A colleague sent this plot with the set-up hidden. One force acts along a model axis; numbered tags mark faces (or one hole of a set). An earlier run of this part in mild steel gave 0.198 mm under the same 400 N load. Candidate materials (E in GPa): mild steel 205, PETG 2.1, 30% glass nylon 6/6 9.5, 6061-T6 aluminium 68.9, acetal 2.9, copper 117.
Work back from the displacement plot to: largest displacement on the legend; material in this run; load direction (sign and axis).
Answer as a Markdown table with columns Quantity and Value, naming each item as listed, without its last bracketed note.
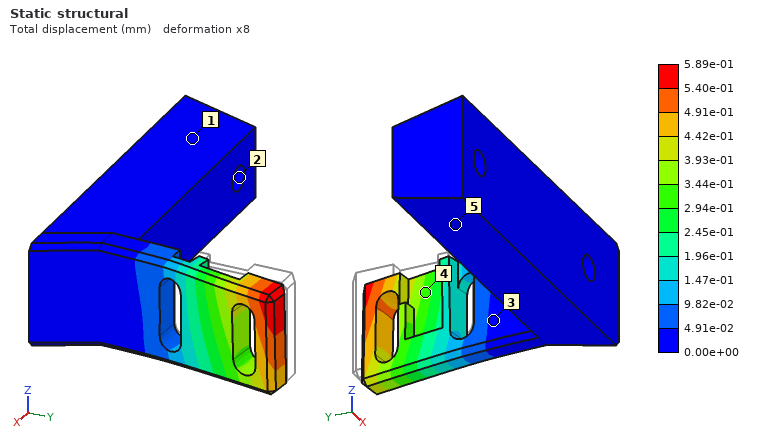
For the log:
| Quantity | Value |
|---|---|
| largest displacement on the legend | 5.89e-01 mm |
| material in this run | 6061-T6 aluminium |
| load direction | +X |
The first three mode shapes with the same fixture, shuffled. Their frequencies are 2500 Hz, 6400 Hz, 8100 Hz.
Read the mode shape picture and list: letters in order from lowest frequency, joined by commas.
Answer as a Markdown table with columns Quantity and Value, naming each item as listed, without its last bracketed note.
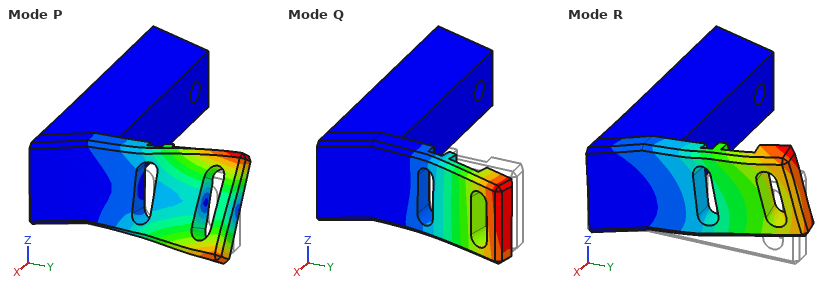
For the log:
| Quantity | Value |
|---|---|
| letters in order from lowest frequency, joined by commas | Q, R, P |
